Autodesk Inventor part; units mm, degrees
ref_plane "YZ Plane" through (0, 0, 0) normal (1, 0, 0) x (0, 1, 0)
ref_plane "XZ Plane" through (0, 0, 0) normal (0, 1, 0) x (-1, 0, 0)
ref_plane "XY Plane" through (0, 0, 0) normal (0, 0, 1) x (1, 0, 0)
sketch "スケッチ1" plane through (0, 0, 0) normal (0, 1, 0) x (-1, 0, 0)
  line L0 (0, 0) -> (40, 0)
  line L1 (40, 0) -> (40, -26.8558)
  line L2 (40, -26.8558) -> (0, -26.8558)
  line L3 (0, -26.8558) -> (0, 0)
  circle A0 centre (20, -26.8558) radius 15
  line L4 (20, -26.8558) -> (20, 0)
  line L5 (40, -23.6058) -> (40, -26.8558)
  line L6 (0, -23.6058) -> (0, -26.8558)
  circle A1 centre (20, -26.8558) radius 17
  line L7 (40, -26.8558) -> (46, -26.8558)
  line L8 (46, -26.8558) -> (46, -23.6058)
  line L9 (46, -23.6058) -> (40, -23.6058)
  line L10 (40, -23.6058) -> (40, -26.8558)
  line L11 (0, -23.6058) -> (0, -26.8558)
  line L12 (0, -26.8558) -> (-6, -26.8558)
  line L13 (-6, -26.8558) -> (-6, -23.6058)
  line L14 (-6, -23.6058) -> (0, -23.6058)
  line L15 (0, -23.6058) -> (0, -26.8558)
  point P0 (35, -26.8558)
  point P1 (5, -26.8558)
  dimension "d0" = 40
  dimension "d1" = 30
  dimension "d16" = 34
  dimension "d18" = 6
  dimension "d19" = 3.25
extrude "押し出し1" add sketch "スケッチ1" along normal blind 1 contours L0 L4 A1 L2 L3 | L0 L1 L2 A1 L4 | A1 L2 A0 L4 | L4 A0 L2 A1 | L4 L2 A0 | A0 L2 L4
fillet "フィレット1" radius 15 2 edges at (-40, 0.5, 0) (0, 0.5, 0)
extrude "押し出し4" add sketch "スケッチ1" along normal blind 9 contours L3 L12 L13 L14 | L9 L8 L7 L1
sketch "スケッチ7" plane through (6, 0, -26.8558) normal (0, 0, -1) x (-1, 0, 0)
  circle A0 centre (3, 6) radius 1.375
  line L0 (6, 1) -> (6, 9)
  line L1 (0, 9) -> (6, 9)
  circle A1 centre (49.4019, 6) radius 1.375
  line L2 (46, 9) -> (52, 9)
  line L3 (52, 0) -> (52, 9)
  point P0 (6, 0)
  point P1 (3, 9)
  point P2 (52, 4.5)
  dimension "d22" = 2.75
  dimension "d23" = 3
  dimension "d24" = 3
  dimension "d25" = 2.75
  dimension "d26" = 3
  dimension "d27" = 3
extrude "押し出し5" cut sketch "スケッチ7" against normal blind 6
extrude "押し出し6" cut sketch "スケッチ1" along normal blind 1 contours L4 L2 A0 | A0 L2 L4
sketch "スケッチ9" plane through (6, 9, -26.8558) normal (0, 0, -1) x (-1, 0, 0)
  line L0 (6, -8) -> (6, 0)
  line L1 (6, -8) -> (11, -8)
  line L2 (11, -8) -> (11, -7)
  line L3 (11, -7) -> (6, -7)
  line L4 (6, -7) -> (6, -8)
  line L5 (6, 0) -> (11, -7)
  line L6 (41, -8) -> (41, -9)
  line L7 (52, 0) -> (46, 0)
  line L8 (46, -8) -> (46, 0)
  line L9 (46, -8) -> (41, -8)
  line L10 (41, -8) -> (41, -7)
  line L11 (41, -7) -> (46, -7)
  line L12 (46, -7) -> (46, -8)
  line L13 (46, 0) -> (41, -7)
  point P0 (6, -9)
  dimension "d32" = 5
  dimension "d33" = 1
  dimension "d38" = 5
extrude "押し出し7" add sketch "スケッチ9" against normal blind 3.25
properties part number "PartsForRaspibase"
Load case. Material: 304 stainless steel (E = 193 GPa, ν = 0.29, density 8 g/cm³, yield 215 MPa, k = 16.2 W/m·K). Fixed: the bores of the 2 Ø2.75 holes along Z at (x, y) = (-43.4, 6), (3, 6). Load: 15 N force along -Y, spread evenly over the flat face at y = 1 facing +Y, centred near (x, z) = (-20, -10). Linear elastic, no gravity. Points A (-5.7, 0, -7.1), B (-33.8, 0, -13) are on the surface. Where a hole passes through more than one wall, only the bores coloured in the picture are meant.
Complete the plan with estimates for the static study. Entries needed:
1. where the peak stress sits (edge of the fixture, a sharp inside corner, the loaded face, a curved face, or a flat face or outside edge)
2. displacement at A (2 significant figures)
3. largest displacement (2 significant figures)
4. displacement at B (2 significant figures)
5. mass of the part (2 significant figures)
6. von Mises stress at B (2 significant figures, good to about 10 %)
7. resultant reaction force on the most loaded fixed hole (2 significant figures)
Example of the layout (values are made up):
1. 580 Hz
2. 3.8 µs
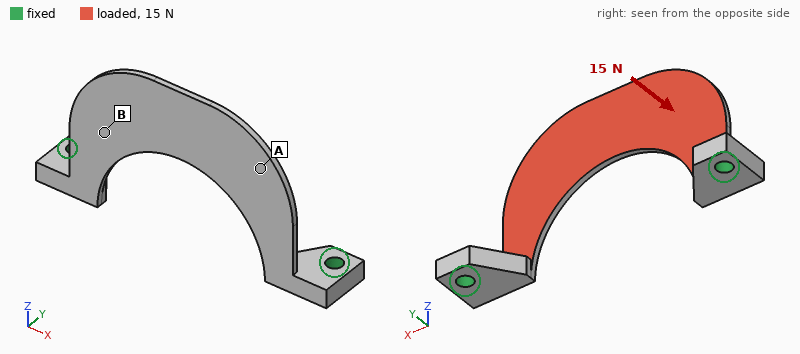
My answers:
1. a curved face
2. 0.098 mm
3. 0.17 mm
4. 0.055 mm
5. 8.7 g
6. 17 MPa
7. 7.5 N
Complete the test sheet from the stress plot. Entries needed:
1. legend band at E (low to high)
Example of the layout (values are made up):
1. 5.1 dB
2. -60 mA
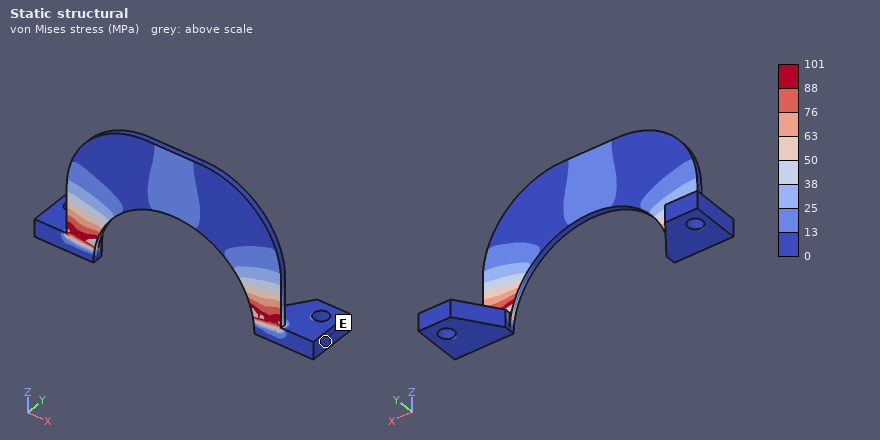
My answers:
1. 0 to 13 MPa
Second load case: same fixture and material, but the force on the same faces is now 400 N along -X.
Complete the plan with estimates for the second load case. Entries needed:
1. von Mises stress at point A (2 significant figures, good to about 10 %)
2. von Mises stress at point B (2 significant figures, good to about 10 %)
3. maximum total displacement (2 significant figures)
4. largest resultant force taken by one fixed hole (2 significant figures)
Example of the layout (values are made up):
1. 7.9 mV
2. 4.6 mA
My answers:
1. 27 MPa
2. 12 MPa
3. 39 µm
4. 240 N
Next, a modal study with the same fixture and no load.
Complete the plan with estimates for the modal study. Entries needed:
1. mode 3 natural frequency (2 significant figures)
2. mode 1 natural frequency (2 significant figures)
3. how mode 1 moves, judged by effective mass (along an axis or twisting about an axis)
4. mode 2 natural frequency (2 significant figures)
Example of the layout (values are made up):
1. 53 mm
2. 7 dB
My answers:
1. 5700 Hz
2. 870 Hz
3. along Y
4. 2600 Hz
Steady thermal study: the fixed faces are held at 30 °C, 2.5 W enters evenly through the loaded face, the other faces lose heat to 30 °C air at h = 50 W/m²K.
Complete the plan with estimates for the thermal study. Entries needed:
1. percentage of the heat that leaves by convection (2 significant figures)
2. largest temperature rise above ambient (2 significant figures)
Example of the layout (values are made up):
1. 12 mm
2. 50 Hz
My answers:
1. 69 %
2. 55 K
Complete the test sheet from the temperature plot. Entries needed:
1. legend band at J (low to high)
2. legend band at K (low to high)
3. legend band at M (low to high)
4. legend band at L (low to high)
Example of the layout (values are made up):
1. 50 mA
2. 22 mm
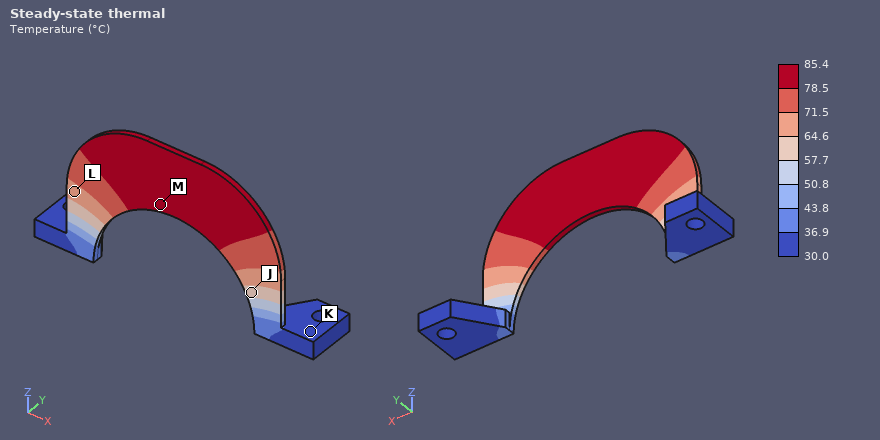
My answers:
1. 57.7 to 64.6 °C
2. 30.0 to 36.9 °C
3. 78.5 to 85.4 °C
4. 64.6 to 71.5 °C
